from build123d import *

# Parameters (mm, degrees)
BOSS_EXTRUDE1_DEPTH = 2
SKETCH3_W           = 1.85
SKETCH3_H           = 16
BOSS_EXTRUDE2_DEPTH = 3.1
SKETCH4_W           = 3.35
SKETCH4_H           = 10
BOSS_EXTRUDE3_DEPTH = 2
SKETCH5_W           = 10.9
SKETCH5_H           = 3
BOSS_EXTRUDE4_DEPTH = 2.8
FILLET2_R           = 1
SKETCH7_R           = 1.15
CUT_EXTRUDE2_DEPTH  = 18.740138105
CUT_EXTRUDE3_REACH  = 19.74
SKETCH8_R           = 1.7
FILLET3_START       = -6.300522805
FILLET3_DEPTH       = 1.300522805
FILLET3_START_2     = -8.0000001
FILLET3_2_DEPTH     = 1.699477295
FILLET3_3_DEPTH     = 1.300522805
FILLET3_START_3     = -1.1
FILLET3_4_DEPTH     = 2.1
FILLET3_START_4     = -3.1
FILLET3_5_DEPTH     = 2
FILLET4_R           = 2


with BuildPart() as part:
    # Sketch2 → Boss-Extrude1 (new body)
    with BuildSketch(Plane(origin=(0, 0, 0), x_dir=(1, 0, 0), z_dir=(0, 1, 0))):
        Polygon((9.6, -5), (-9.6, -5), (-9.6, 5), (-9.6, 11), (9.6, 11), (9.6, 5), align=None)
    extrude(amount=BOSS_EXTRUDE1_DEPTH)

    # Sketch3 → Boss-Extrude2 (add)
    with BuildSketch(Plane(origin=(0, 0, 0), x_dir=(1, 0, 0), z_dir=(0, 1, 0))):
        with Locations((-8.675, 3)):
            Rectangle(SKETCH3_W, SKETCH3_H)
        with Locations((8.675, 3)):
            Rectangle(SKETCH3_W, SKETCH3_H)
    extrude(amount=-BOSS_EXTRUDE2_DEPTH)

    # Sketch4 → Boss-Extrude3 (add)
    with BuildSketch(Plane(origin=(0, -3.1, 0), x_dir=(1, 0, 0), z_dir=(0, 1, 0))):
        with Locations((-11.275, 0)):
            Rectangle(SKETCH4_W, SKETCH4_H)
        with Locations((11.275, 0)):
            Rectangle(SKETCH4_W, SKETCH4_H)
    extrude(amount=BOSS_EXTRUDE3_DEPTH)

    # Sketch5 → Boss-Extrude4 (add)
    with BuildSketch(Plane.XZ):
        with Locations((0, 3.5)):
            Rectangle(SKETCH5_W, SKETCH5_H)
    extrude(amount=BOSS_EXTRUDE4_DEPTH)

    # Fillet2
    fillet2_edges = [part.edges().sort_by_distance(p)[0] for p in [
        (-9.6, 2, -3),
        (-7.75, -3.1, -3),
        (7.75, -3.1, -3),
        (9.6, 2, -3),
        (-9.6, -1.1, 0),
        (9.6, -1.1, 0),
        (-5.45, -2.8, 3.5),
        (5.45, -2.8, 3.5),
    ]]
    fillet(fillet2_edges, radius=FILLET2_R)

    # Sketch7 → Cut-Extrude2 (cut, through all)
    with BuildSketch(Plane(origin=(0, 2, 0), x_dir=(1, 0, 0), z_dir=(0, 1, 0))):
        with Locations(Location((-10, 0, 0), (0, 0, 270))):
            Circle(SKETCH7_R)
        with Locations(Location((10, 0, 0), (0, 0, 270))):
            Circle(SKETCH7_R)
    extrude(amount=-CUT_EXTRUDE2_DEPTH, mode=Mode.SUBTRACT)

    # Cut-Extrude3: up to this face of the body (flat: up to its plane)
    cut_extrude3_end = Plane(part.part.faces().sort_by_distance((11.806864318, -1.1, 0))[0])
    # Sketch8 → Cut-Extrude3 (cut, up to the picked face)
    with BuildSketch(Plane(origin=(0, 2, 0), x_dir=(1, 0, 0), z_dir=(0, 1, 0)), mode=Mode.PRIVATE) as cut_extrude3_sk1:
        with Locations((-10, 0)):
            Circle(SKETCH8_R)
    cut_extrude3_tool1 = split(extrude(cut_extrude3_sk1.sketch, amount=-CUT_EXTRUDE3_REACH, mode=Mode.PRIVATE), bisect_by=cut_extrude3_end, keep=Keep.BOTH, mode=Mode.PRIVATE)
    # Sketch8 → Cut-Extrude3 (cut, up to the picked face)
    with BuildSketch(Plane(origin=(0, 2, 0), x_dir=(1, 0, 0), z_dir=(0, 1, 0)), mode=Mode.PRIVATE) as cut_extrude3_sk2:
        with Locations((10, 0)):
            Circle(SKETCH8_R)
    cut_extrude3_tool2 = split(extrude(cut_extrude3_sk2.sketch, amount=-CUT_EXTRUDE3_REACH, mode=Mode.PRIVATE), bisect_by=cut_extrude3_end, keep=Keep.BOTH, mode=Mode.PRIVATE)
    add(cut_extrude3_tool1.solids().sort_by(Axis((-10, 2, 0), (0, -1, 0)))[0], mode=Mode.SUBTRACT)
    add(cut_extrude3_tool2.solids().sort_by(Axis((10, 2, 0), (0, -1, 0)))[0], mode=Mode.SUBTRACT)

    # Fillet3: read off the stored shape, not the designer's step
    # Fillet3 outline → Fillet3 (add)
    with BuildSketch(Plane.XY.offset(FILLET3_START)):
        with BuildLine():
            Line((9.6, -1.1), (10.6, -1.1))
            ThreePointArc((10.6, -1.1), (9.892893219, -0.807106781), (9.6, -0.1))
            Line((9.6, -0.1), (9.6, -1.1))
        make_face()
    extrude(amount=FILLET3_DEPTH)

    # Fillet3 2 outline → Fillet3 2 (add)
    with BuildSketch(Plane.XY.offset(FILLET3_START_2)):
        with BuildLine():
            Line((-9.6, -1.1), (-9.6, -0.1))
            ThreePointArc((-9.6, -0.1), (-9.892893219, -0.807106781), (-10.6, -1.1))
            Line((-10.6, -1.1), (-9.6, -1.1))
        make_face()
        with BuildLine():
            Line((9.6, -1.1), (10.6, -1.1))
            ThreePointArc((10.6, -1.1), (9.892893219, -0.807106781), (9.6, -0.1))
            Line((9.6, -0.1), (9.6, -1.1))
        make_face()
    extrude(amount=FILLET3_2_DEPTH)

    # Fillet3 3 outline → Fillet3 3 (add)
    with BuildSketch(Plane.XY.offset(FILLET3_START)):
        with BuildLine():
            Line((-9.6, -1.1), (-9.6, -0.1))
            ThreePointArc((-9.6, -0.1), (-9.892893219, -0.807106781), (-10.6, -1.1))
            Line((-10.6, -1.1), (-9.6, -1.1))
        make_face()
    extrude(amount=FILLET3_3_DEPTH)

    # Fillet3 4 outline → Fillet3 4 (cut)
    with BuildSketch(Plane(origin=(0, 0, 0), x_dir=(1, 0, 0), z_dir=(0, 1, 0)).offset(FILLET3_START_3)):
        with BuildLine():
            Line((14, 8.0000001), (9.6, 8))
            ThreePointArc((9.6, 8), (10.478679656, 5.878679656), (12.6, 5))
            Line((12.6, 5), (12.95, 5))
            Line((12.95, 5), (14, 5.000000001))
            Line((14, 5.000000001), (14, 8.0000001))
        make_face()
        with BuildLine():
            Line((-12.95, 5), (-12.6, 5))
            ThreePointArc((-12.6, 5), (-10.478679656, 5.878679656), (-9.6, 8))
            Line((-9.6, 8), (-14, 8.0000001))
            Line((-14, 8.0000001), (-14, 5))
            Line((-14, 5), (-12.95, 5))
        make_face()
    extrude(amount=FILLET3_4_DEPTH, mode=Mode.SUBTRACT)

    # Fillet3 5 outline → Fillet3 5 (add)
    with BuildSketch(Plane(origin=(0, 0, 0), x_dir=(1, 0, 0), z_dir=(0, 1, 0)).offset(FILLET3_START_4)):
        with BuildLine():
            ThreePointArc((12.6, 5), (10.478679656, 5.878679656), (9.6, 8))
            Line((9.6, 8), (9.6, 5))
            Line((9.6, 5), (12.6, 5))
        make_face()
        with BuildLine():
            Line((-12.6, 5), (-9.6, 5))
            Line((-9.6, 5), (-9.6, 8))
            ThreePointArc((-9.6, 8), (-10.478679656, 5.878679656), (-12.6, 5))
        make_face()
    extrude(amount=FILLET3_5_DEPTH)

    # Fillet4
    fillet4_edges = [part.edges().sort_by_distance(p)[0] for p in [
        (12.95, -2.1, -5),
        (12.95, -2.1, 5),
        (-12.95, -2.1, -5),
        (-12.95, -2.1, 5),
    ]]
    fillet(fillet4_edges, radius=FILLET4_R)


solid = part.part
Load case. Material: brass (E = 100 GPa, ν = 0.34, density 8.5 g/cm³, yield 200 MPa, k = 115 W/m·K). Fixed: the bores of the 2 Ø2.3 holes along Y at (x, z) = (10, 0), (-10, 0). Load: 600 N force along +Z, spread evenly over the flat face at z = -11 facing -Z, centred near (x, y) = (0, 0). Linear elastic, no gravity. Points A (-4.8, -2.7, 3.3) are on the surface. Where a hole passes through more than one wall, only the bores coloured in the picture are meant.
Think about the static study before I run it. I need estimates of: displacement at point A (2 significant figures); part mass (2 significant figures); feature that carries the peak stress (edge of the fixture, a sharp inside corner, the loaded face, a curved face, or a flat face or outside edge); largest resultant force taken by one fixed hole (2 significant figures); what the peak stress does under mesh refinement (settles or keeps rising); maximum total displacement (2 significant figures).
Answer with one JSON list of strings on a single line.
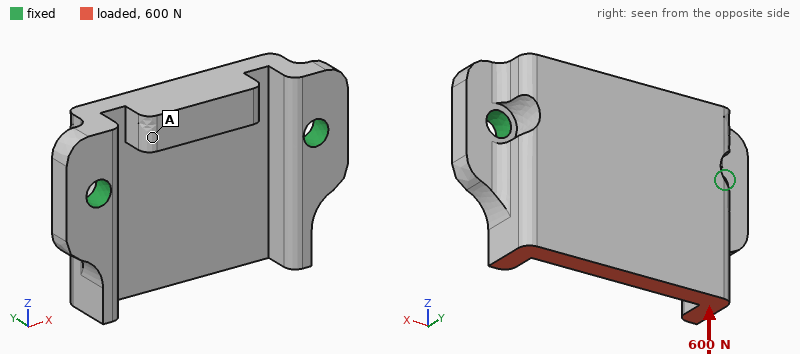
["3.8 µm", "8.3 g", "edge of the fixture", "300 N", "keeps rising", "21 µm"]
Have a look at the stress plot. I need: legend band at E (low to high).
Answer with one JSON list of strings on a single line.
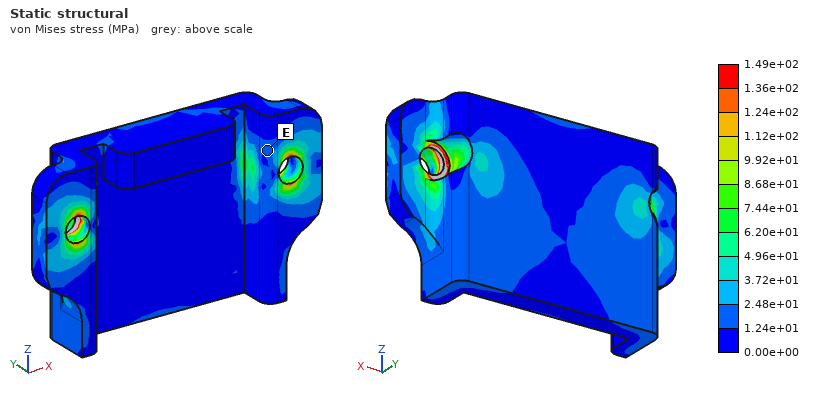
["1.24e+01 to 2.48e+01 MPa"]
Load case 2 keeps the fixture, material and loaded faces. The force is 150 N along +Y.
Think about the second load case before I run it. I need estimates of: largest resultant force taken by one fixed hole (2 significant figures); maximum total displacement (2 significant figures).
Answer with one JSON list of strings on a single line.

["98 N", "33 µm"]
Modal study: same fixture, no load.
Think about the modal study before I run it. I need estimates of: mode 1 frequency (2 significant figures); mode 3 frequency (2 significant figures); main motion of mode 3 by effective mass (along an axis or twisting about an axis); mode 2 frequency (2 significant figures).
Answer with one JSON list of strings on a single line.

["9100 Hz", "18 kHz", "along Y", "15 kHz"]
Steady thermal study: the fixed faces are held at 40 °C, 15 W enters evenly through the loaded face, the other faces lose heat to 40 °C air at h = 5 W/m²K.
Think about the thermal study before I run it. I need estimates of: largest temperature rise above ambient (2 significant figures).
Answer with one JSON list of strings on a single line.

["39 K"]
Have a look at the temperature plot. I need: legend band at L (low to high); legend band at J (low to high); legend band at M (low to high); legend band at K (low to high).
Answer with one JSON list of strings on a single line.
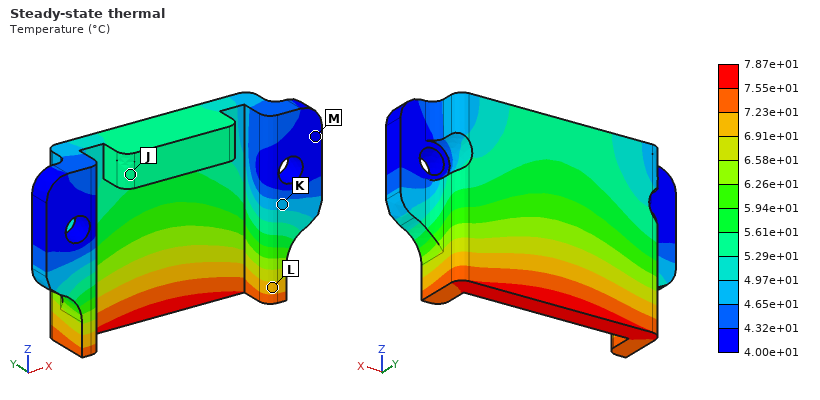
["6.91e+01 to 7.23e+01 °C", "5.29e+01 to 5.61e+01 °C", "4.00e+01 to 4.32e+01 °C", "4.65e+01 to 4.97e+01 °C"]
